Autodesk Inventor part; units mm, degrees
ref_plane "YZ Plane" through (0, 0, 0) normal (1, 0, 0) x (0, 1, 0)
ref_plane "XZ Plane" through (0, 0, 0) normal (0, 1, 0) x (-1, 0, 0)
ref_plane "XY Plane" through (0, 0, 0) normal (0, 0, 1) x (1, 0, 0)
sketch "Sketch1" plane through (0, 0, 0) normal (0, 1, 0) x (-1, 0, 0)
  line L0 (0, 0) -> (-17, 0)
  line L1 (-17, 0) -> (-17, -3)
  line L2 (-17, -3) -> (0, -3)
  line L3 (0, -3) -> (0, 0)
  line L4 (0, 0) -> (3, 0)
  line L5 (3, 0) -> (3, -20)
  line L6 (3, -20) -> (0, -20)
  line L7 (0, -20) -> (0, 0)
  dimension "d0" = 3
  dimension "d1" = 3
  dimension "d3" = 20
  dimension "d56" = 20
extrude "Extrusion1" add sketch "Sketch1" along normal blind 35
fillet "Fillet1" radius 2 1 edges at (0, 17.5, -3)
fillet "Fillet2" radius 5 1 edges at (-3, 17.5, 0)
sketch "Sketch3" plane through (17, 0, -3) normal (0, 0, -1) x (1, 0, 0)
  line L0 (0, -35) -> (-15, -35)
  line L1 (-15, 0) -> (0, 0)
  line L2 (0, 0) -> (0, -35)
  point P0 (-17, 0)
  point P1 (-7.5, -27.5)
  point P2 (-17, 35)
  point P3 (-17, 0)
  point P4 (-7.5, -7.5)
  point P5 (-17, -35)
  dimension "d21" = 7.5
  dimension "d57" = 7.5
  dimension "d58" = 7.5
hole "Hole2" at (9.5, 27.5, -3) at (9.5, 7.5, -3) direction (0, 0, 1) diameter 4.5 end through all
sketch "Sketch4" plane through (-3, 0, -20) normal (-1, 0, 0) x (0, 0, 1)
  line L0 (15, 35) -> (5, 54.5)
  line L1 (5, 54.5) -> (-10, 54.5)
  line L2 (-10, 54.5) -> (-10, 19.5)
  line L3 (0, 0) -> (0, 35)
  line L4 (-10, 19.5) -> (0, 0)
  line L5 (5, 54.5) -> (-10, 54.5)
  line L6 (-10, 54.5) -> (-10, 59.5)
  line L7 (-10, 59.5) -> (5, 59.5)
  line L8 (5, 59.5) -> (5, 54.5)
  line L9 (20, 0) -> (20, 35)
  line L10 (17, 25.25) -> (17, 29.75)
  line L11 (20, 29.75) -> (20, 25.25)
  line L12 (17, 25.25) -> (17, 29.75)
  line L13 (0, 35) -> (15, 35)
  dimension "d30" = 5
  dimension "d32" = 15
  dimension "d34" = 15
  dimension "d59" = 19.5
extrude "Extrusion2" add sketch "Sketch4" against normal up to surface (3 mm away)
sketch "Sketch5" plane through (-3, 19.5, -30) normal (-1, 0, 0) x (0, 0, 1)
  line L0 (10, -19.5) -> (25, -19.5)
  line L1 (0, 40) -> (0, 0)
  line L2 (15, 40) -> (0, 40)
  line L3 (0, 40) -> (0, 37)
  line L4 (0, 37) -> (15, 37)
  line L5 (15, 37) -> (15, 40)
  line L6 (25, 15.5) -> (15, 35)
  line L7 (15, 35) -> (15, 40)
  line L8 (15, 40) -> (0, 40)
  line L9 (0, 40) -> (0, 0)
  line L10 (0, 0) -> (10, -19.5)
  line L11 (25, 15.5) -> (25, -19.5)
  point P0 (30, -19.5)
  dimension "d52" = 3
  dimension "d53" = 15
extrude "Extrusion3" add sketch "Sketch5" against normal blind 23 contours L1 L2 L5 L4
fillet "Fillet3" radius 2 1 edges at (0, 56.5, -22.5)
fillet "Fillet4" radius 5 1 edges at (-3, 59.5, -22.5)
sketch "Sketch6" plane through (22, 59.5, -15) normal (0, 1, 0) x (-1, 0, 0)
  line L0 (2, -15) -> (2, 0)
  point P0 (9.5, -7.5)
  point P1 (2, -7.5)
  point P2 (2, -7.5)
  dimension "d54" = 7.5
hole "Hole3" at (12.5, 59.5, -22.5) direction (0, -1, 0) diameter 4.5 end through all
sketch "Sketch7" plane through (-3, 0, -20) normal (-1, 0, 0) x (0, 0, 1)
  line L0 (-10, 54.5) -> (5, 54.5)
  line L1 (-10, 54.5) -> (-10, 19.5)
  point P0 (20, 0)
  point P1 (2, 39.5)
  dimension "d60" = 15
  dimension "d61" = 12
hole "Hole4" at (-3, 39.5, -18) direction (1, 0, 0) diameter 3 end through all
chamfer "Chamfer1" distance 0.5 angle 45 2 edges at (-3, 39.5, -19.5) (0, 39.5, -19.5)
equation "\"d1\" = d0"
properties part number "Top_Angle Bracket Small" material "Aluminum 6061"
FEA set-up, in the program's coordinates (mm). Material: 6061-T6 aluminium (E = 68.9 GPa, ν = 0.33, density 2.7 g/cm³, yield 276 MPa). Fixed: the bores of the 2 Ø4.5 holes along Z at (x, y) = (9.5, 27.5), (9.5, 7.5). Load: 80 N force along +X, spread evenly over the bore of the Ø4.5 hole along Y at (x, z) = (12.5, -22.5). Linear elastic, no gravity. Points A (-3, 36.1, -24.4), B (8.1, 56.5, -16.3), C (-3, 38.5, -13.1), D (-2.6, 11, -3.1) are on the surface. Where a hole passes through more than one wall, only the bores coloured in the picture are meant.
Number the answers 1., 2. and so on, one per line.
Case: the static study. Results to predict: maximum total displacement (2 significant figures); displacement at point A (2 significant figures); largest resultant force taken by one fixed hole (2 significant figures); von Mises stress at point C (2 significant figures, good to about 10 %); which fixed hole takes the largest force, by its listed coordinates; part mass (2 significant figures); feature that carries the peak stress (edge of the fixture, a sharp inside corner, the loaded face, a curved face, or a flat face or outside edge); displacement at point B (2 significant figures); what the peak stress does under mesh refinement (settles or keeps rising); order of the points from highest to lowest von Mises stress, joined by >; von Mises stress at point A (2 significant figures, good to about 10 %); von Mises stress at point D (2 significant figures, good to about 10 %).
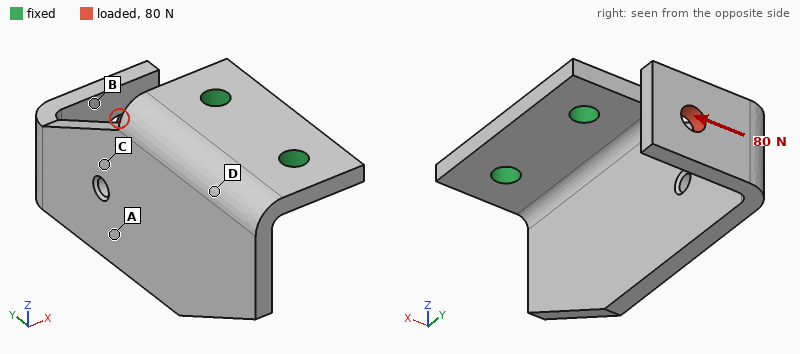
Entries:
1. 0.70 mm
2. 0.22 mm
3. 180 N
4. 62 MPa
5. (9.5, 27.5)
6. 18 g
7. a sharp inside corner
8. 0.43 mm
9. keeps rising
10. C > A > D > B
11. 48 MPa
12. 19 MPa
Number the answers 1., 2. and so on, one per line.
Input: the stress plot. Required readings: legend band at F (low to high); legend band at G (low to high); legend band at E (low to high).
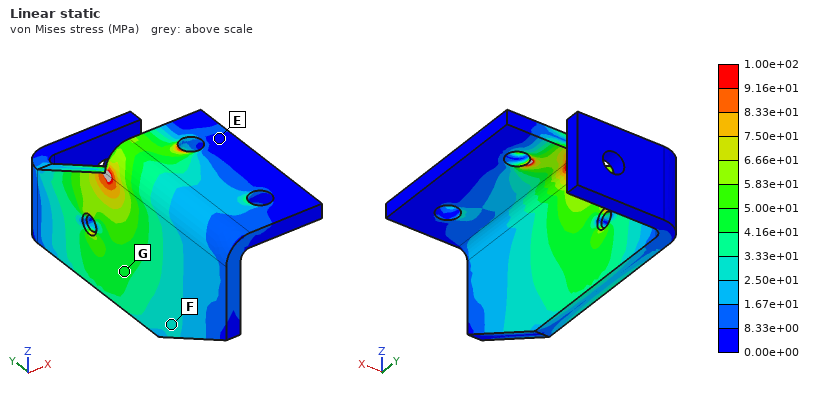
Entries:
1. 2.50e+01 to 3.33e+01 MPa
2. 4.16e+01 to 5.00e+01 MPa
3. 0.00e+00 to 8.33e+00 MPa
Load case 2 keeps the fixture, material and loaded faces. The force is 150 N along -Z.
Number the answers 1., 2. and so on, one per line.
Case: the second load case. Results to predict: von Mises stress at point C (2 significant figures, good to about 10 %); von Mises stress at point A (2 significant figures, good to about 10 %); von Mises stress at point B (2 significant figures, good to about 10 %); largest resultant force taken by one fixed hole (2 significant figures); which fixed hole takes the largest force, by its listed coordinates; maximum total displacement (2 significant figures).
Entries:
1. 59 MPa
2. 49 MPa
3. 13 MPa
4. 340 N
5. (9.5, 27.5)
6. 0.61 mm
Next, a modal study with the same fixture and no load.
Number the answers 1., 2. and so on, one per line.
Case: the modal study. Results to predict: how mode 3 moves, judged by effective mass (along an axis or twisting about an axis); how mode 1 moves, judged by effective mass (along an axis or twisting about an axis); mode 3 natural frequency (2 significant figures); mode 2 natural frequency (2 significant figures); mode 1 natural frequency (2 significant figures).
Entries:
1. along Z
2. along X
3. 2500 Hz
4. 1900 Hz
5. 950 Hz
